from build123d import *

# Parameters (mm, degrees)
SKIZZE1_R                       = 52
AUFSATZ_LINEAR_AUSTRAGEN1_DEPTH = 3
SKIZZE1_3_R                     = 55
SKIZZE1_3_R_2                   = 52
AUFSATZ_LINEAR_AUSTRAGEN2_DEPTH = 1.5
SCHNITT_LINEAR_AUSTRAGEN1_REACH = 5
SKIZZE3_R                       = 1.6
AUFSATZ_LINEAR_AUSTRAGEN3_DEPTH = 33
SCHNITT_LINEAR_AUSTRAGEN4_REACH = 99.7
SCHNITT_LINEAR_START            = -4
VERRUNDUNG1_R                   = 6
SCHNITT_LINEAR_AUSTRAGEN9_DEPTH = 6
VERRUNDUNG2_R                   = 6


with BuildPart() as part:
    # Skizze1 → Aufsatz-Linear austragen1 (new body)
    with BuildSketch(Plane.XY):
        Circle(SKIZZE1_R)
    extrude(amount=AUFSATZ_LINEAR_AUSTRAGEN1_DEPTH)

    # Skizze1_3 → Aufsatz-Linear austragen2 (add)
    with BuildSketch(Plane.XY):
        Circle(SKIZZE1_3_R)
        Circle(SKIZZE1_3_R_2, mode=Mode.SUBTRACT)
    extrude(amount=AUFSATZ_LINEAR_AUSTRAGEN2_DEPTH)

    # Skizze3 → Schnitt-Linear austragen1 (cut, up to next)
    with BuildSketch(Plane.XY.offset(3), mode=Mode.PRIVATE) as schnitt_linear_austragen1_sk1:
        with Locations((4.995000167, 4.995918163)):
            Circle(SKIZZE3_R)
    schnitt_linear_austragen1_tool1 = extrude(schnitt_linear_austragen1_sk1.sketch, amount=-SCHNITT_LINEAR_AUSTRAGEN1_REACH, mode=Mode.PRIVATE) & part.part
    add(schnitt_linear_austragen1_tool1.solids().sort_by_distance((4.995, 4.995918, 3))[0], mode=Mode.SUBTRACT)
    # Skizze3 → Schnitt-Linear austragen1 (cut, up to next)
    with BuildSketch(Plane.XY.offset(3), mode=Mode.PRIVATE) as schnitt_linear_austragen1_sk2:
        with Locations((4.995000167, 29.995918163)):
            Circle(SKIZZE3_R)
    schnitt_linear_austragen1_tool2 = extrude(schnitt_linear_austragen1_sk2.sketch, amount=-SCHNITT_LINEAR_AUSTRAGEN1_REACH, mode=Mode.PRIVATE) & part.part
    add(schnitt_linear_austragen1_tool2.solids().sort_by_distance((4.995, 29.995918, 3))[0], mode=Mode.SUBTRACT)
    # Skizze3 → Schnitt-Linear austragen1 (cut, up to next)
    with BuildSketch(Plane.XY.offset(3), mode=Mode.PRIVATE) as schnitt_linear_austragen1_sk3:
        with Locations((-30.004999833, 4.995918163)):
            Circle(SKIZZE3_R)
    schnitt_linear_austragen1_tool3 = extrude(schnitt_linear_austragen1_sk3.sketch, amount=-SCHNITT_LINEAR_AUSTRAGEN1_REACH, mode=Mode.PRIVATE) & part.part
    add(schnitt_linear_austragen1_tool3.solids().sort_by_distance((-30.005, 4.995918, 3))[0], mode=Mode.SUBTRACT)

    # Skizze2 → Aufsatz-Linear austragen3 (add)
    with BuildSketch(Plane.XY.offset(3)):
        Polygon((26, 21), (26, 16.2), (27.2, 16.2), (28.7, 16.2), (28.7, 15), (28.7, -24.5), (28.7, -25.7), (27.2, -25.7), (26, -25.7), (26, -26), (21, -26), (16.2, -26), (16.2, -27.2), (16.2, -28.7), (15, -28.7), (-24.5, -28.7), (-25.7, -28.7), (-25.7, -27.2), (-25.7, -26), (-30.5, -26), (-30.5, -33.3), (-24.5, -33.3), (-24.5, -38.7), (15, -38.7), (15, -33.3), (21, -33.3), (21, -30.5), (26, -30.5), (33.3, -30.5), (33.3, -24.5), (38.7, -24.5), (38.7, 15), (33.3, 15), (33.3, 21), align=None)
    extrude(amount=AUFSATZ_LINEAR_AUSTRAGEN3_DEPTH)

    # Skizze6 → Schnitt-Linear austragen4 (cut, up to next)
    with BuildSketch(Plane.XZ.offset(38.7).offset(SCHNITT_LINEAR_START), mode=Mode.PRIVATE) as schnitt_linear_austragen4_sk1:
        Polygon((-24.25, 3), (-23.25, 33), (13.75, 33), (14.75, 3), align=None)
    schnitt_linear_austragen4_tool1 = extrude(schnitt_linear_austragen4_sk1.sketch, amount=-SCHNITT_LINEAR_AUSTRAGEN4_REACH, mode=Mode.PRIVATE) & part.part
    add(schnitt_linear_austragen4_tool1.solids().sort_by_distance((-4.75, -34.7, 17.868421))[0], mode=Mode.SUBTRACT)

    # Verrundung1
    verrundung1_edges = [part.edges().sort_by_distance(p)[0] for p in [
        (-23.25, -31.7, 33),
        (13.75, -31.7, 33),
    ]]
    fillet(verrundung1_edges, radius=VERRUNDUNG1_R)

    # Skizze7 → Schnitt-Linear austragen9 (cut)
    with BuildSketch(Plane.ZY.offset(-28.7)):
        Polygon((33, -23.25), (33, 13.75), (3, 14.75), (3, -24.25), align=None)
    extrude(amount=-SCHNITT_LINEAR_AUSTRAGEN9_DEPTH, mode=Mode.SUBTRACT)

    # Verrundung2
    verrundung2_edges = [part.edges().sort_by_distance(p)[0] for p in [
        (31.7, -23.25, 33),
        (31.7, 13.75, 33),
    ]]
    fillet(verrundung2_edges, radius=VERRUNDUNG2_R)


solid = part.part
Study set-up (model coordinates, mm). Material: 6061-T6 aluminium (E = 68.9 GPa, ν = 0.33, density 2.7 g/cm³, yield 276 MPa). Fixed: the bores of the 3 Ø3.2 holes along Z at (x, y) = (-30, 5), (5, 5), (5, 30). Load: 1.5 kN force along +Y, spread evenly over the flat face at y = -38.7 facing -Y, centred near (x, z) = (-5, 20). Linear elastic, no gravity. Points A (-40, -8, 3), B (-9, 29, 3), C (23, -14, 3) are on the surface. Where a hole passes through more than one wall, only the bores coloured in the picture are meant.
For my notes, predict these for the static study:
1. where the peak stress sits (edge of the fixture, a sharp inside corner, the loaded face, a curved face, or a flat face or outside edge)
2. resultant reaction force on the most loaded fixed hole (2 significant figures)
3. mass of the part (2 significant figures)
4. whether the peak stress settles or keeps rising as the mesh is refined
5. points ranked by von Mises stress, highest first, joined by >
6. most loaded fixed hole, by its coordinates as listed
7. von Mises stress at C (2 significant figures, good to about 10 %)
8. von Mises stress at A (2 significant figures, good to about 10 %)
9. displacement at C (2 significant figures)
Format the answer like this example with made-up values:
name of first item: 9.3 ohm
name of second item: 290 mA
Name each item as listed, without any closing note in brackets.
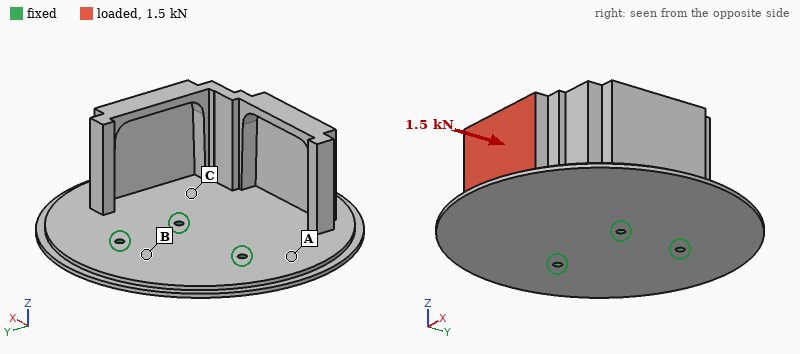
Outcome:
where the peak stress sits: edge of the fixture
resultant reaction force on the most loaded fixed hole: 960 N
mass of the part: 120 g
whether the peak stress settles or keeps rising as the mesh is refined: keeps rising
points ranked by von Mises stress, highest first, joined by >: A > C > B
most loaded fixed hole, by its coordinates as listed: (5, 5)
von Mises stress at C: 43 MPa
von Mises stress at A: 81 MPa
displacement at C: 0.39 mm
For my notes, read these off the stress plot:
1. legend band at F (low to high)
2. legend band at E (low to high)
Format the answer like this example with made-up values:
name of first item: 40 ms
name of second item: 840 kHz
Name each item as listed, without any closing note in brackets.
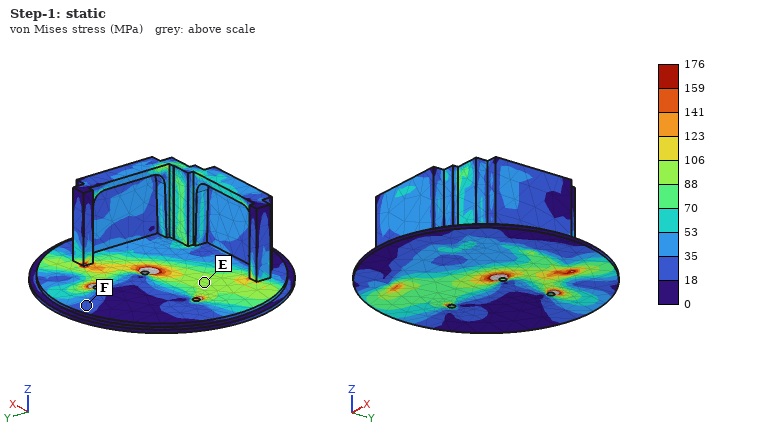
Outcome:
legend band at F: 18 to 35 MPa
legend band at E: 88 to 106 MPa
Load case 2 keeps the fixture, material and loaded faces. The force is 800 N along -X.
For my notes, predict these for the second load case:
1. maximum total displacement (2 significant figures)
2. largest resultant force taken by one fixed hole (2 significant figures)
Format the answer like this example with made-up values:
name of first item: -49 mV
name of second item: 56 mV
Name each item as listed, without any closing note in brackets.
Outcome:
maximum total displacement: 0.52 mm
largest resultant force taken by one fixed hole: 930 N
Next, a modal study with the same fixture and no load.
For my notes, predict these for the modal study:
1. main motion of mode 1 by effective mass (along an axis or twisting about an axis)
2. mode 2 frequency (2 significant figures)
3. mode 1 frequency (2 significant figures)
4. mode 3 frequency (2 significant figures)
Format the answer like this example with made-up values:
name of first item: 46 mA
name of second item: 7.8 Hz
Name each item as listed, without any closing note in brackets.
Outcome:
main motion of mode 1 by effective mass: along Z
mode 2 frequency: 780 Hz
mode 1 frequency: 540 Hz
mode 3 frequency: 1800 Hz
